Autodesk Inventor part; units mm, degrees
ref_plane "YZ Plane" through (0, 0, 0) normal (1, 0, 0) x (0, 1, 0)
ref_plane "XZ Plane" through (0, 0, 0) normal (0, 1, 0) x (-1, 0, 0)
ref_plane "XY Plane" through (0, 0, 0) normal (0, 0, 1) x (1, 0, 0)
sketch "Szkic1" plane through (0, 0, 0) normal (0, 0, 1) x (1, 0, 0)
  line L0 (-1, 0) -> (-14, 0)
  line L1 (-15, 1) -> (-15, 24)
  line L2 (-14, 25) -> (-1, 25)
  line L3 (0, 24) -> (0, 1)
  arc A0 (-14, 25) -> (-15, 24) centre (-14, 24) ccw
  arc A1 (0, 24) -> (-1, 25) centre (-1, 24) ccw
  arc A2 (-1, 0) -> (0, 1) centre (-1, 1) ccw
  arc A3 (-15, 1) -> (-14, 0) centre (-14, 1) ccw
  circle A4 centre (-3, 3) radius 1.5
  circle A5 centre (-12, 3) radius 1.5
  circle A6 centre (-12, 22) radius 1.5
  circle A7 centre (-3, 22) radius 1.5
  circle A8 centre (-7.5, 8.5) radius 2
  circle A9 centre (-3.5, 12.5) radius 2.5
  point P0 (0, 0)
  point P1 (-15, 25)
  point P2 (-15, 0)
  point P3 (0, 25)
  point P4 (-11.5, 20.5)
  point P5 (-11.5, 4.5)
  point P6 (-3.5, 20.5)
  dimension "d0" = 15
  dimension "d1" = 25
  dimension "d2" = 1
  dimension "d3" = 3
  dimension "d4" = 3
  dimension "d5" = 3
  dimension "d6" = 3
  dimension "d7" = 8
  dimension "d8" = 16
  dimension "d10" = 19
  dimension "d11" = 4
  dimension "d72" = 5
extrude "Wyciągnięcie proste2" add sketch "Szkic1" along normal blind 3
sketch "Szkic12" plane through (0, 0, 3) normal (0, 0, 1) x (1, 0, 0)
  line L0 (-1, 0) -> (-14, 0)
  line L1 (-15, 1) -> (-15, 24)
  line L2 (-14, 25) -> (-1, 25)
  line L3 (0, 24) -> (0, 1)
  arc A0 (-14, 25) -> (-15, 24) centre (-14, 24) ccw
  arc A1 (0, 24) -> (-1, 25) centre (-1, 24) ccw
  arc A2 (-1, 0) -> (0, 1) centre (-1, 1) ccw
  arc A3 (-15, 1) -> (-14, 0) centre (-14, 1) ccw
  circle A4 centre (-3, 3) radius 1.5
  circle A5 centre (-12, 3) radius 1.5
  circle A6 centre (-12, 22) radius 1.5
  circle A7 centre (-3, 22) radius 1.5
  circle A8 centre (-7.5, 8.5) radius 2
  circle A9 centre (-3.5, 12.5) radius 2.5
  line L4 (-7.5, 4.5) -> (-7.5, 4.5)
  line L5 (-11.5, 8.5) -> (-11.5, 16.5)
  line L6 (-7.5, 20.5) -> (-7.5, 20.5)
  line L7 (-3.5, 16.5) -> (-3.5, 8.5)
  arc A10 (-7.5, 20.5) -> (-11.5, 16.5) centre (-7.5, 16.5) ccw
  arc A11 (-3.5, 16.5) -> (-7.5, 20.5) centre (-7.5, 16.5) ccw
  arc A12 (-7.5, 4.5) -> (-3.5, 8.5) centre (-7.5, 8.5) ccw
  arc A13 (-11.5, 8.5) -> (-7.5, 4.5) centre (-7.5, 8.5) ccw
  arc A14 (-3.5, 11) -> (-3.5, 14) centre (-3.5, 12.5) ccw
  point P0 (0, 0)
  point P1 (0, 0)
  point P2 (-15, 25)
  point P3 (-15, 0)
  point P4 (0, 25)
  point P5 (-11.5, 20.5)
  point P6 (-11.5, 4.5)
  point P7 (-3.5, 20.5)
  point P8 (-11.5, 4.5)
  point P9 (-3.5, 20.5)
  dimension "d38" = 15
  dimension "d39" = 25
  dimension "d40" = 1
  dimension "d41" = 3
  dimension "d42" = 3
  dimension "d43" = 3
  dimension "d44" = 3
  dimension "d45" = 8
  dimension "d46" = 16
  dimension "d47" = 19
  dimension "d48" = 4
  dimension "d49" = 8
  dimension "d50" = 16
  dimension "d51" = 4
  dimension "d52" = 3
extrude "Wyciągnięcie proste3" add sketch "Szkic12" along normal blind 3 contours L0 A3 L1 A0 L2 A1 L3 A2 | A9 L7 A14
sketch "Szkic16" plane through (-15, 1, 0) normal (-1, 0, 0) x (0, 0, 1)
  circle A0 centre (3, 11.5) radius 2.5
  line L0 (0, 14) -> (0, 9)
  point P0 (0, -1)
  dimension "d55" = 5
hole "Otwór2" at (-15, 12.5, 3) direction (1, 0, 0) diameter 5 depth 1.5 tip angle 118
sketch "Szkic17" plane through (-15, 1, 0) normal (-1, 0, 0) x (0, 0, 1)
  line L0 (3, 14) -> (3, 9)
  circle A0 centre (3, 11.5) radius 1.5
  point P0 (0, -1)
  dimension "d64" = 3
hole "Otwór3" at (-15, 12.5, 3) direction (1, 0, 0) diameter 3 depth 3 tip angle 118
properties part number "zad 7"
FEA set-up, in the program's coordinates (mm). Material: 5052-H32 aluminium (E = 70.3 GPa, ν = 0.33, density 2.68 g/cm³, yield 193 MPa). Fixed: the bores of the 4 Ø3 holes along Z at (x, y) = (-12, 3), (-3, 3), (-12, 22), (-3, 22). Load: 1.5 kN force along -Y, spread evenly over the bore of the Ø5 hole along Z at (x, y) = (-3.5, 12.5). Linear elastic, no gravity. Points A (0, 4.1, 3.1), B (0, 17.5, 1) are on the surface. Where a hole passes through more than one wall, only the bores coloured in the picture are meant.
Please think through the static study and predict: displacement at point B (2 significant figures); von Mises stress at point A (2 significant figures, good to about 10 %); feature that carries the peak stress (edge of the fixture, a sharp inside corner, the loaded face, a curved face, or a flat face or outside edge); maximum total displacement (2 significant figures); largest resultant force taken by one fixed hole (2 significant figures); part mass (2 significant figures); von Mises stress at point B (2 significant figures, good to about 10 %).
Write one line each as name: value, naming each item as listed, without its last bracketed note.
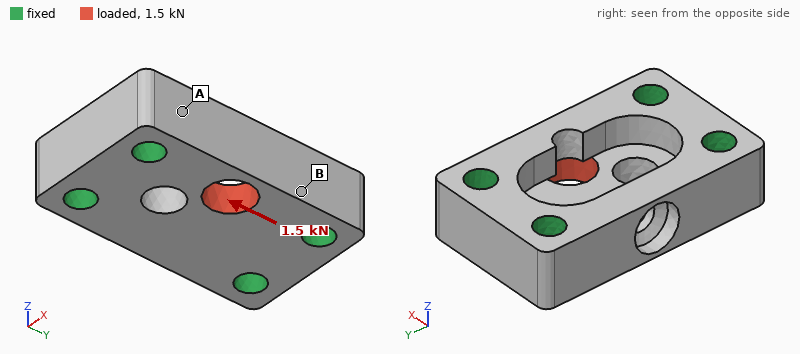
displacement at point B: 1.7 µm
von Mises stress at point A: 11 MPa
feature that carries the peak stress: a curved face
maximum total displacement: 4.0 µm
largest resultant force taken by one fixed hole: 630 N
part mass: 4.2 g
von Mises stress at point B: 23 MPa
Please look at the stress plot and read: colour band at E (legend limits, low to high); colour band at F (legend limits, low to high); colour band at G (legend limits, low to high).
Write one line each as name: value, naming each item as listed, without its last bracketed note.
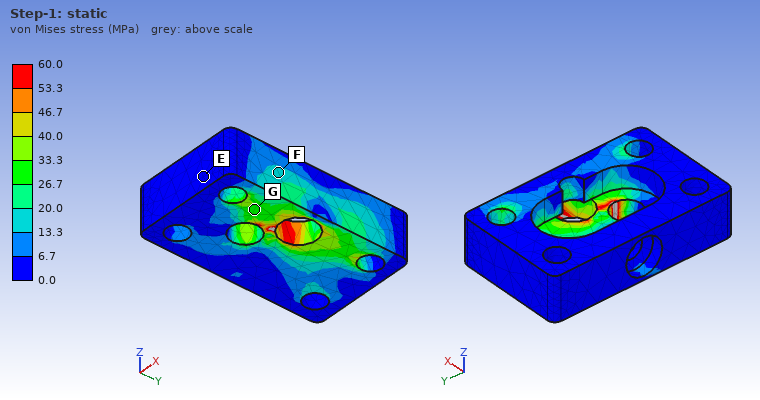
colour band at E: 0.0 to 6.7 MPa
colour band at F: 13.3 to 20.0 MPa
colour band at G: 26.7 to 33.3 MPa
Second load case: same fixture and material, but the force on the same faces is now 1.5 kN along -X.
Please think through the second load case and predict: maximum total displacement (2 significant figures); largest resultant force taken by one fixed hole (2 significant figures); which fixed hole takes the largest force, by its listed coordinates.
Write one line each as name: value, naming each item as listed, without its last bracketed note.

maximum total displacement: 16 µm
largest resultant force taken by one fixed hole: 560 N
which fixed hole takes the largest force, by its listed coordinates: (-12, 22)
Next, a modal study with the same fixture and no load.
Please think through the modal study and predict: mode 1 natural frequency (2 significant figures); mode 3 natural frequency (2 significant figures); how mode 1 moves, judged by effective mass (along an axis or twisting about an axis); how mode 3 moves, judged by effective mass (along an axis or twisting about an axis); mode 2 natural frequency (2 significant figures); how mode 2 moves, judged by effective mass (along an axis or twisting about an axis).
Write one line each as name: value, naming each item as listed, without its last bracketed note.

mode 1 natural frequency: 66 kHz
mode 3 natural frequency: 80 kHz
how mode 1 moves, judged by effective mass: along Z
how mode 3 moves, judged by effective mass: along X
mode 2 natural frequency: 73 kHz
how mode 2 moves, judged by effective mass: along X
